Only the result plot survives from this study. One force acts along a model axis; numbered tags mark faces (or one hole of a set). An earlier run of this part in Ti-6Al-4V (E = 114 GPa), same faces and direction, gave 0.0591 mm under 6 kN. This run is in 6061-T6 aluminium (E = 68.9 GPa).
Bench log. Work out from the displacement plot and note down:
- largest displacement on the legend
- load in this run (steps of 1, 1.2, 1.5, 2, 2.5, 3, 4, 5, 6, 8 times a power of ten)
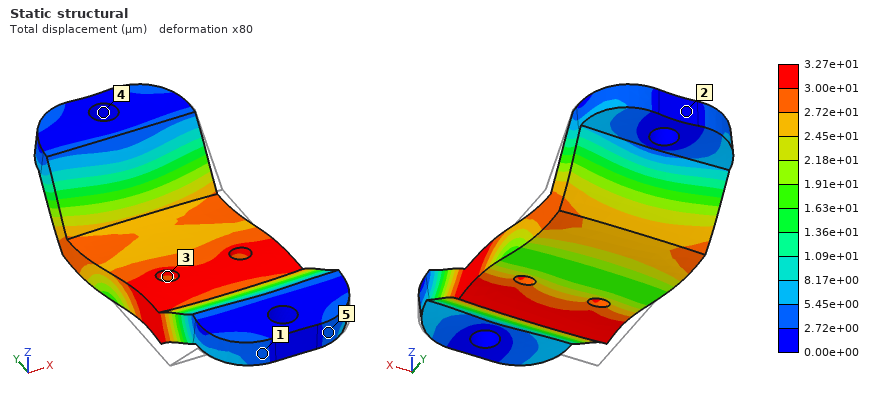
3.27e+01 µm
2 kN
